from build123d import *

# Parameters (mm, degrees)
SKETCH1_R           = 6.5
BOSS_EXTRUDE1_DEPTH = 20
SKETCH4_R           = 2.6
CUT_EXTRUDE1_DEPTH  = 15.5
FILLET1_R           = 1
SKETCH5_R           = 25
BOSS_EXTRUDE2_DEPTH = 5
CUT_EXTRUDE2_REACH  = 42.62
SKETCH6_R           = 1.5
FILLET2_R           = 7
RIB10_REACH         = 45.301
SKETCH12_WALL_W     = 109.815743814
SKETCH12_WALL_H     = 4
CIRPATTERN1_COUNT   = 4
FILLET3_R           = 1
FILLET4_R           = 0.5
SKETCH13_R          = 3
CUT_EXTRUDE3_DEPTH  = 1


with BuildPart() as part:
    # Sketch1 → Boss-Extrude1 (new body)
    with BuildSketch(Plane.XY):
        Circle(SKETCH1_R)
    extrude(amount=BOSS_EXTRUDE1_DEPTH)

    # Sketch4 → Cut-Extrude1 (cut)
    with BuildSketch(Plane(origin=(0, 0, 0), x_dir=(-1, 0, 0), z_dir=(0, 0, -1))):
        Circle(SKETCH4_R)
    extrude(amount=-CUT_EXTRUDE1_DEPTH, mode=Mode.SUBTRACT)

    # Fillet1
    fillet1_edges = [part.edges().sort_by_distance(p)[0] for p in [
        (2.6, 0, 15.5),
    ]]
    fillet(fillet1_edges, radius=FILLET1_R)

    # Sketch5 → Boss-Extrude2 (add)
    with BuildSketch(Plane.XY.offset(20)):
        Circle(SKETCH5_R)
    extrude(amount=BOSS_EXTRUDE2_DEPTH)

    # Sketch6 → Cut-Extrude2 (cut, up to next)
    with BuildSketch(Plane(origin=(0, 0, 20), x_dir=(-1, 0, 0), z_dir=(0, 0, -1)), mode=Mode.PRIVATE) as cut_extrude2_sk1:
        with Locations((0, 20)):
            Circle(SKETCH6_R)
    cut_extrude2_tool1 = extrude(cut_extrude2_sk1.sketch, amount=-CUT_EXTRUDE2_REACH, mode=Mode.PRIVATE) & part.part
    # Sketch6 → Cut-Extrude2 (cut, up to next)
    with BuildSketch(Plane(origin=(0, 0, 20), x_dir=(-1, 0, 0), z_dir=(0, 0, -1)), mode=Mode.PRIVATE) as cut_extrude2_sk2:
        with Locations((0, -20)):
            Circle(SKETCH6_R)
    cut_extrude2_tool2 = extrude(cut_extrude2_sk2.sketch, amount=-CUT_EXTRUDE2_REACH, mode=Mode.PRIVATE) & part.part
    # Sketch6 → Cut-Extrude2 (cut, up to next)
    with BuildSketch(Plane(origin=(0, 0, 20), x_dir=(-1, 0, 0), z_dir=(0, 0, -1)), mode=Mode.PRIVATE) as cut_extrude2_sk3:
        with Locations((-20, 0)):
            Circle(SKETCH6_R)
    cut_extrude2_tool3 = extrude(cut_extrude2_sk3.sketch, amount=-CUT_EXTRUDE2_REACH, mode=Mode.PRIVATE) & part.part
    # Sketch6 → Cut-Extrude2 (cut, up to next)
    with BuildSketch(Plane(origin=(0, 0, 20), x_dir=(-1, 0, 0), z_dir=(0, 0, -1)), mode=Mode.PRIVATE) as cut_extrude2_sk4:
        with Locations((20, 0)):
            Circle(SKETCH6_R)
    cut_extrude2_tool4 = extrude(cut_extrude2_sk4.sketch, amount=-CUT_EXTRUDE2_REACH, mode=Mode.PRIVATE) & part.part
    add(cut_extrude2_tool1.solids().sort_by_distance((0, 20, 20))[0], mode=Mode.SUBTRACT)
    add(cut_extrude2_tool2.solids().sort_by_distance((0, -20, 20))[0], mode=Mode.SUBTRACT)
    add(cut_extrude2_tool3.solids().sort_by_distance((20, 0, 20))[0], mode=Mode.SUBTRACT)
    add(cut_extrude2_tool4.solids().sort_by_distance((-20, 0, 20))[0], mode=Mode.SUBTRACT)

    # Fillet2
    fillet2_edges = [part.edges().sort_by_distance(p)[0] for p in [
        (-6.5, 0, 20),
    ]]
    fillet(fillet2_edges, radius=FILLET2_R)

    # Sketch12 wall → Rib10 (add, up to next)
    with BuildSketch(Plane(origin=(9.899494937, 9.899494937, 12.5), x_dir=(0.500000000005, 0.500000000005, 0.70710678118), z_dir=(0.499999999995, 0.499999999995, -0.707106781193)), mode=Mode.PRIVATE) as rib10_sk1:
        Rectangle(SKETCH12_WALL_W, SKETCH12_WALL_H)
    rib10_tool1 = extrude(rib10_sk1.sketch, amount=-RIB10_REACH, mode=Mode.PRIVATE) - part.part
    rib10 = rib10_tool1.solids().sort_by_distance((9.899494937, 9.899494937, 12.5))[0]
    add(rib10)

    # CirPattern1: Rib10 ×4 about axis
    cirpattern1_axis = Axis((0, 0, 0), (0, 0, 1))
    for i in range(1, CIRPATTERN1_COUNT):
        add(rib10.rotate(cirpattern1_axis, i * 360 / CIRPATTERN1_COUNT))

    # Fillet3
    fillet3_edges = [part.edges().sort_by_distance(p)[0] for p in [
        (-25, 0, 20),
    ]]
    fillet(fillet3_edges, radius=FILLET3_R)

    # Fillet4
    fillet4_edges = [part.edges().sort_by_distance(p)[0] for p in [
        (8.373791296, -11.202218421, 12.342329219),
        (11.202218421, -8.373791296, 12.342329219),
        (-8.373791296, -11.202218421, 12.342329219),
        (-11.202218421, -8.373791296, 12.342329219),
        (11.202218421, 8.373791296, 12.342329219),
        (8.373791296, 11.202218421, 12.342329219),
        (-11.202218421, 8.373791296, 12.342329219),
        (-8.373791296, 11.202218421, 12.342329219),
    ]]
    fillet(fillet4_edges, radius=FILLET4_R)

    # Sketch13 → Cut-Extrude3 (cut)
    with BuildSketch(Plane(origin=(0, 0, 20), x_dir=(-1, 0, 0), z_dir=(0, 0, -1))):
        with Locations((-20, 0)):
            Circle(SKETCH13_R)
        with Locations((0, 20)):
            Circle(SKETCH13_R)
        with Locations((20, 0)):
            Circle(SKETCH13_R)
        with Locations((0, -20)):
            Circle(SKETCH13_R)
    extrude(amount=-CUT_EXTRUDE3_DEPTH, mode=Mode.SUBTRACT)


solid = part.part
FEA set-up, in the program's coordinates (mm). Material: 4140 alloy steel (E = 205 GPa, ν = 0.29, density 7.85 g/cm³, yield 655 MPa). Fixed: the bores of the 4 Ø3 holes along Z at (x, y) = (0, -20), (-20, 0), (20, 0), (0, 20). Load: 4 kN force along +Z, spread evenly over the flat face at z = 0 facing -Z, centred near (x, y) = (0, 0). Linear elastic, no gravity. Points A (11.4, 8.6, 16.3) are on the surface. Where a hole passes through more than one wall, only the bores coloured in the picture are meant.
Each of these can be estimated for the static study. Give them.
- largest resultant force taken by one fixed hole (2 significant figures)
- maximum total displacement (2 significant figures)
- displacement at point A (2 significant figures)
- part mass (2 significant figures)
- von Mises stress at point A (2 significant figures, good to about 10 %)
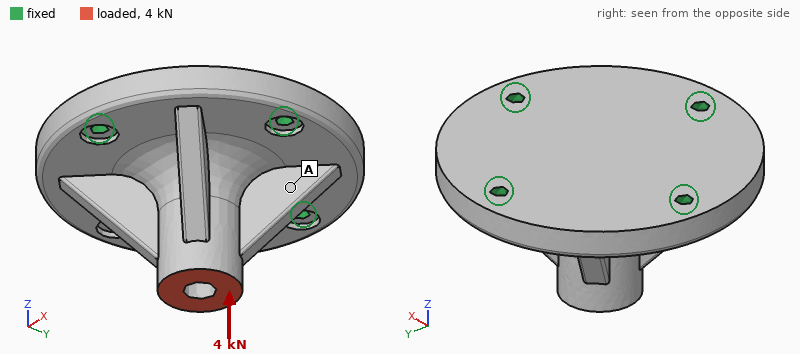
1.1 kN
8.2 µm
5.1 µm
110 g
20 MPa
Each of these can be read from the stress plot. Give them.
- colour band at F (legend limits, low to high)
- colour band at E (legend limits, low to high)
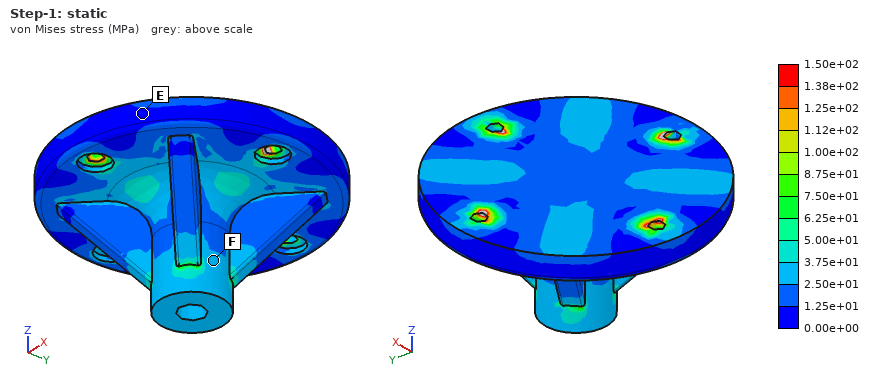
2.50e+01 to 3.75e+01 MPa
0.00e+00 to 1.25e+01 MPa
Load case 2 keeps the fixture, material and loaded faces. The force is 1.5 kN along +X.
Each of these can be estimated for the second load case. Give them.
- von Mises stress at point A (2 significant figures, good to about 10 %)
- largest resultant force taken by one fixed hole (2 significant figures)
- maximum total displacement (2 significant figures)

28 MPa
1.0 kN
14 µm
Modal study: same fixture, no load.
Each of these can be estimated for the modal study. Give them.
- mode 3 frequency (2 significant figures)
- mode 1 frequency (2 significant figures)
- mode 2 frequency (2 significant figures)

16 kHz
16 kHz
16 kHz
